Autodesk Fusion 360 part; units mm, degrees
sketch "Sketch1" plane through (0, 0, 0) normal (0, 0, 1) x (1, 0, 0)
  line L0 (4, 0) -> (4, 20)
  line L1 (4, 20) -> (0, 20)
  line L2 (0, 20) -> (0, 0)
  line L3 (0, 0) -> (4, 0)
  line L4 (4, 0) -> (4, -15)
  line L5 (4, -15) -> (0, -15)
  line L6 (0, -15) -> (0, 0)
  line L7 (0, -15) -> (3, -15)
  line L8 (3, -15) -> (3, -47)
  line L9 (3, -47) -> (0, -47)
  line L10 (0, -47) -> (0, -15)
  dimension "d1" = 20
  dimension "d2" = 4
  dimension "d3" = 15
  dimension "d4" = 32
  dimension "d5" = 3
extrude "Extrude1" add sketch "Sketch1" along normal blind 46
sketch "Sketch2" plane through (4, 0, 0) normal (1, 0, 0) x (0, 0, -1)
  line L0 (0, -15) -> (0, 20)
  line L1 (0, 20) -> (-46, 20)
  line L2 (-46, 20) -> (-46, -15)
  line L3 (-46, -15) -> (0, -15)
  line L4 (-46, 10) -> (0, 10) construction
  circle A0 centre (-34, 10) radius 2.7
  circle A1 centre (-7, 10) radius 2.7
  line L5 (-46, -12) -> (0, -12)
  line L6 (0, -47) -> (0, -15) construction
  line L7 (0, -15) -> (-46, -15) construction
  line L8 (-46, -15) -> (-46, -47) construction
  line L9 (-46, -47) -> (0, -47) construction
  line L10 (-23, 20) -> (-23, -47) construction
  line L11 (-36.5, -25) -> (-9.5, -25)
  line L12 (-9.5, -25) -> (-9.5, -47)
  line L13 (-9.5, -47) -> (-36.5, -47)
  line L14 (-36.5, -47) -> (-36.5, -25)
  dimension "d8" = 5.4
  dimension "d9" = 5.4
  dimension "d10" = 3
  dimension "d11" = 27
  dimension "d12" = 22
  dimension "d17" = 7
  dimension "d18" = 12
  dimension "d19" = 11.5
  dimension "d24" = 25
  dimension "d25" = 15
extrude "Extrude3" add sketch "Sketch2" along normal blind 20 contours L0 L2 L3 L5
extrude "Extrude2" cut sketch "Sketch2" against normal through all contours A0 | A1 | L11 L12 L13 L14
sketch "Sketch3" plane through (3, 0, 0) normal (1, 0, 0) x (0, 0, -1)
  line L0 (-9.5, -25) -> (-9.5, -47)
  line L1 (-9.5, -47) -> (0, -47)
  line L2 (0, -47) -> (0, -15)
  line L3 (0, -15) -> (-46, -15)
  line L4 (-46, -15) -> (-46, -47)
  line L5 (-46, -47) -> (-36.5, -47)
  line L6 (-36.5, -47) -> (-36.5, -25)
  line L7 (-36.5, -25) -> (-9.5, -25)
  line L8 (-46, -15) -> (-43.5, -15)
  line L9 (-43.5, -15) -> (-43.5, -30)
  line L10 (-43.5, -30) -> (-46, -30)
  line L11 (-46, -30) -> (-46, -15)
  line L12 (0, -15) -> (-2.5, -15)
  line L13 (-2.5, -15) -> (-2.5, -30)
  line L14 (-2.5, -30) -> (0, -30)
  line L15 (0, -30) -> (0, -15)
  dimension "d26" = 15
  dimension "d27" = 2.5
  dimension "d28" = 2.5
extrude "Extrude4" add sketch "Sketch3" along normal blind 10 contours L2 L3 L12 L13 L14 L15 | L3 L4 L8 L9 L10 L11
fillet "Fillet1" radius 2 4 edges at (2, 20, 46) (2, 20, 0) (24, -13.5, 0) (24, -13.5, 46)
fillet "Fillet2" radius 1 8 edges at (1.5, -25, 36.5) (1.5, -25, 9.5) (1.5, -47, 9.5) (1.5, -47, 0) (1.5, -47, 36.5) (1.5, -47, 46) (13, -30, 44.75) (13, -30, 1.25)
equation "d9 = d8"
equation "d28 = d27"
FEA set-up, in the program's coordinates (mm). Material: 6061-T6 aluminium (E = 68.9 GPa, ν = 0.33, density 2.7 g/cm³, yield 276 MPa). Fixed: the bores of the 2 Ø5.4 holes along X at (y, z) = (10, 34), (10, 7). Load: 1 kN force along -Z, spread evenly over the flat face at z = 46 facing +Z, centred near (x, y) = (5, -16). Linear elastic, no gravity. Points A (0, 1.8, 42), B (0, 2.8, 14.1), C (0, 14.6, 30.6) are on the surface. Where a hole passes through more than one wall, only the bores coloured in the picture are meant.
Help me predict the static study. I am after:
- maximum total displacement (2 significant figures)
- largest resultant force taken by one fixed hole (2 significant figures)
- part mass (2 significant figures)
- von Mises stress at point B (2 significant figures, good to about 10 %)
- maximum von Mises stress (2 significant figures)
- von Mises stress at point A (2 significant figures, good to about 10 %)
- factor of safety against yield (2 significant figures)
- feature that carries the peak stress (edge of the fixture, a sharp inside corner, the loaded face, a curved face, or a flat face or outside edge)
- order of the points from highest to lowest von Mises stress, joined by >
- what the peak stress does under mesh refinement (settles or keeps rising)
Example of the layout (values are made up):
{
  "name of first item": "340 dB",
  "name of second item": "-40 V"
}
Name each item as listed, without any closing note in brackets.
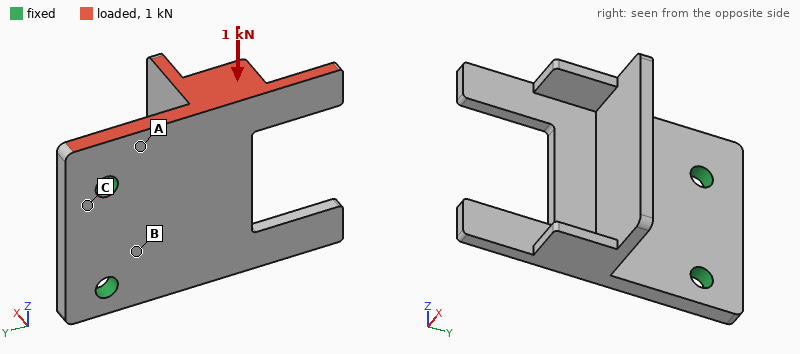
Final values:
{
  "maximum total displacement": "0.11 mm",
  "largest resultant force taken by one fixed hole": "990 N",
  "part mass": "33 g",
  "von Mises stress at point B": "11 MPa",
  "maximum von Mises stress": "160 MPa",
  "von Mises stress at point A": "21 MPa",
  "factor of safety against yield": "1.7",
  "feature that carries the peak stress": "a curved face",
  "order of the points from highest to lowest von Mises stress, joined by >": "A > B > C",
  "what the peak stress does under mesh refinement": "settles"
}
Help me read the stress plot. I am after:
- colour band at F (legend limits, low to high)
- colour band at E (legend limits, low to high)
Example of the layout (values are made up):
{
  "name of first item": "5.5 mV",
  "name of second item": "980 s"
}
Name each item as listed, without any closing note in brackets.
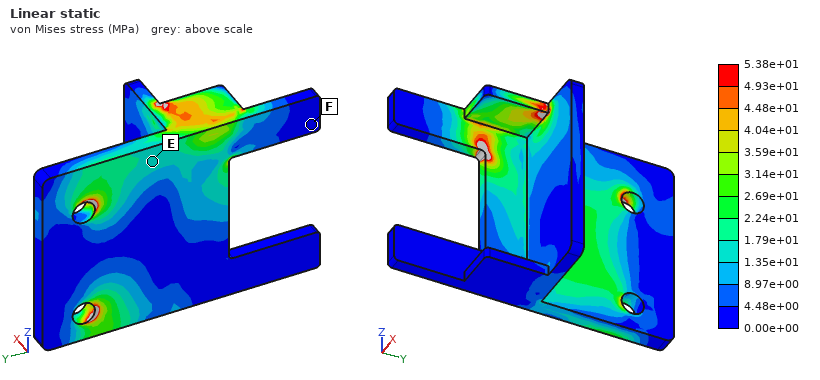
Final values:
{
  "colour band at F": "0.00e+00 to 4.48e+00 MPa",
  "colour band at E": "1.35e+01 to 1.79e+01 MPa"
}
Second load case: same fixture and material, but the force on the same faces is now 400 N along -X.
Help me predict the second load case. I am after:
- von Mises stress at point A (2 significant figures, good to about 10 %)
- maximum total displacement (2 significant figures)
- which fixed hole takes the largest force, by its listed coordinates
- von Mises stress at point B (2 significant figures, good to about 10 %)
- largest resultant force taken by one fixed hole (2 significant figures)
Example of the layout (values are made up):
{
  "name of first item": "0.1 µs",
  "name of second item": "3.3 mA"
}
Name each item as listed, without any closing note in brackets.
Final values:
{
  "von Mises stress at point A": "80 MPa",
  "maximum total displacement": "0.67 mm",
  "which fixed hole takes the largest force, by its listed coordinates": "(10, 34)",
  "von Mises stress at point B": "44 MPa",
  "largest resultant force taken by one fixed hole": "500 N"
}
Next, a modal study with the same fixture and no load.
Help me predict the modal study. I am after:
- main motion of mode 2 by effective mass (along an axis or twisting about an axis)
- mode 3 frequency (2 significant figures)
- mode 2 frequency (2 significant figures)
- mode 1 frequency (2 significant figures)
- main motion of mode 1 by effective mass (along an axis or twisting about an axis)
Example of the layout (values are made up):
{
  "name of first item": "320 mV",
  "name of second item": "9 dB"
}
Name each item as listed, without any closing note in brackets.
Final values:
{
  "main motion of mode 2 by effective mass": "twisting about Y",
  "mode 3 frequency": "5300 Hz",
  "mode 2 frequency": "2200 Hz",
  "mode 1 frequency": "1400 Hz",
  "main motion of mode 1 by effective mass": "along X"
}
